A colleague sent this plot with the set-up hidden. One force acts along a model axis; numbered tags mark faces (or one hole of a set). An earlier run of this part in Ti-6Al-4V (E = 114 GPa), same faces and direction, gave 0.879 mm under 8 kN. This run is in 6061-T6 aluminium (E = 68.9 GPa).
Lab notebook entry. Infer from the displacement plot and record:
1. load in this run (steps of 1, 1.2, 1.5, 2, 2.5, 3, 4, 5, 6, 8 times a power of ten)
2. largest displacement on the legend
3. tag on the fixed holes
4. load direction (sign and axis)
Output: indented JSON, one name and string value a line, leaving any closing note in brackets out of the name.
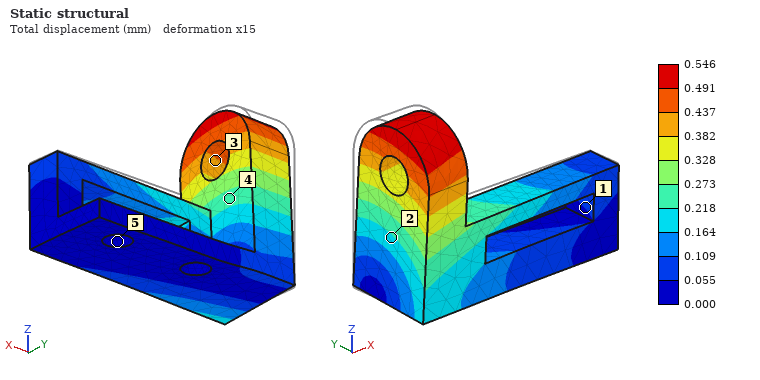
{
  "load in this run": "3 kN",
  "largest displacement on the legend": "0.546 mm",
  "tag on the fixed holes": "5",
  "load direction": "-Y"
}
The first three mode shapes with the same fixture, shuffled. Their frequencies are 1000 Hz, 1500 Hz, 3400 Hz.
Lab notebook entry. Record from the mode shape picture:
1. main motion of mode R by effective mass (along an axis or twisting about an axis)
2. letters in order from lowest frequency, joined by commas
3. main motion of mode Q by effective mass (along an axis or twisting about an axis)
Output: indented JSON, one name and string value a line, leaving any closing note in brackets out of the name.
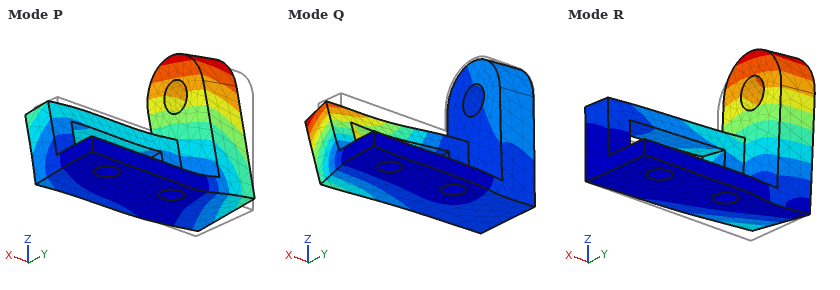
{
  "main motion of mode R by effective mass": "along Y",
  "letters in order from lowest frequency, joined by commas": "R, P, Q",
  "main motion of mode Q by effective mass": "along Z"
}
